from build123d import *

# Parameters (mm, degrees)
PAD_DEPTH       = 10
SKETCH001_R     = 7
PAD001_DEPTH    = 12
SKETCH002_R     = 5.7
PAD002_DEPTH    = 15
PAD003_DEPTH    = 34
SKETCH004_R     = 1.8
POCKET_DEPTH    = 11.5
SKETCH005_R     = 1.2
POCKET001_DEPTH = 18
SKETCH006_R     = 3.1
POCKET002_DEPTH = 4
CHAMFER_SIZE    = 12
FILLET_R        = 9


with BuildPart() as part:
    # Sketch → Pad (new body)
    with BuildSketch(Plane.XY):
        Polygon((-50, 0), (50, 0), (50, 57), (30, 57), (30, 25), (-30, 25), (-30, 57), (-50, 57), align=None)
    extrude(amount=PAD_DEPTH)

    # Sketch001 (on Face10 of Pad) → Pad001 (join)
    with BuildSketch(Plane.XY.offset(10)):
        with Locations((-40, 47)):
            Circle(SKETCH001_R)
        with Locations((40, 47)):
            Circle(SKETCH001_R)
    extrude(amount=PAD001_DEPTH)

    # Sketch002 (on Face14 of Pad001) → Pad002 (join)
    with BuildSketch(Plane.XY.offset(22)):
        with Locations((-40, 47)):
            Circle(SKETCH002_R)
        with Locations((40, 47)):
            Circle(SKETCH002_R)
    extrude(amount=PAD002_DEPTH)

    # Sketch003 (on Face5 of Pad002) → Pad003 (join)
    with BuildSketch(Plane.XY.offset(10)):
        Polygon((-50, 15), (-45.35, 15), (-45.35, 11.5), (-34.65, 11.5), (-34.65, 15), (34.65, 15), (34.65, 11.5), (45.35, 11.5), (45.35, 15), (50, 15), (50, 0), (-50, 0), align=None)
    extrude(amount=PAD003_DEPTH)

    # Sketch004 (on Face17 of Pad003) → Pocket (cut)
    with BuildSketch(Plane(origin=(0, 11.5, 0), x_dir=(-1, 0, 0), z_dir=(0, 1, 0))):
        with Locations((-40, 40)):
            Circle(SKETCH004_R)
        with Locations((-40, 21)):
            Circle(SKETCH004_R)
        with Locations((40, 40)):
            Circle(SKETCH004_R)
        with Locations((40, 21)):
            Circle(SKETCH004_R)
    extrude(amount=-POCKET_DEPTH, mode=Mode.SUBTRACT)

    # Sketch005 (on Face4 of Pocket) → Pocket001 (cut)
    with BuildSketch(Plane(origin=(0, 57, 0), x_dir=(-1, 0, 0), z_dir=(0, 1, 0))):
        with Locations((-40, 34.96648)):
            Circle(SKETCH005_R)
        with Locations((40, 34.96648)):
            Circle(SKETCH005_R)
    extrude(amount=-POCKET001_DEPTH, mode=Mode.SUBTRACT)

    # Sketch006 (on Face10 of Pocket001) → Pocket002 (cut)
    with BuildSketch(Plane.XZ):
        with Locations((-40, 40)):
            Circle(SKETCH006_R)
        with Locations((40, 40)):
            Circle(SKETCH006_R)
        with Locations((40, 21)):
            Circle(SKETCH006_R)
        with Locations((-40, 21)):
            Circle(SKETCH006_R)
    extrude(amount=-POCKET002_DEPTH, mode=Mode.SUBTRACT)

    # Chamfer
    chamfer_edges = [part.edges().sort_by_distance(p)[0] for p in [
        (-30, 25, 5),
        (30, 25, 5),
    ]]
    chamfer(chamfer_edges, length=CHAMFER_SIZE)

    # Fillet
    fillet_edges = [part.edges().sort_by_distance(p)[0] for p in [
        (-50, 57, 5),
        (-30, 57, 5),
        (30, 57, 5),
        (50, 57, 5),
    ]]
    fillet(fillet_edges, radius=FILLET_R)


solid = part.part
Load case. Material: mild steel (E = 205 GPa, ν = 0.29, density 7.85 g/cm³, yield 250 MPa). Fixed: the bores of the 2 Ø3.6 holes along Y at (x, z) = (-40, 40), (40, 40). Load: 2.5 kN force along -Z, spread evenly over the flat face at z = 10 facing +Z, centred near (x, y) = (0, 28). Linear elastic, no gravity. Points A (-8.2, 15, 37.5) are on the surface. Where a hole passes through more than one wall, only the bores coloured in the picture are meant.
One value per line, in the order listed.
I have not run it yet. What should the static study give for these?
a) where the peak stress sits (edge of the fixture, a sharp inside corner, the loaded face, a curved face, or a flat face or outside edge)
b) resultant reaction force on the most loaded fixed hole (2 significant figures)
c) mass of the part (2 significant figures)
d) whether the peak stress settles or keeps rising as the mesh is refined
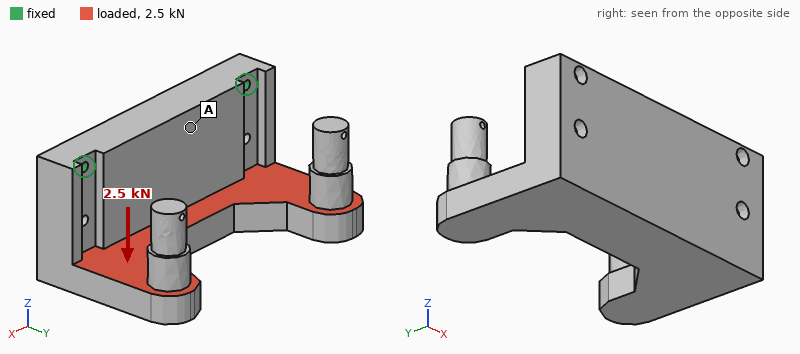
edge of the fixture
1.3 kN
730 g
keeps rising
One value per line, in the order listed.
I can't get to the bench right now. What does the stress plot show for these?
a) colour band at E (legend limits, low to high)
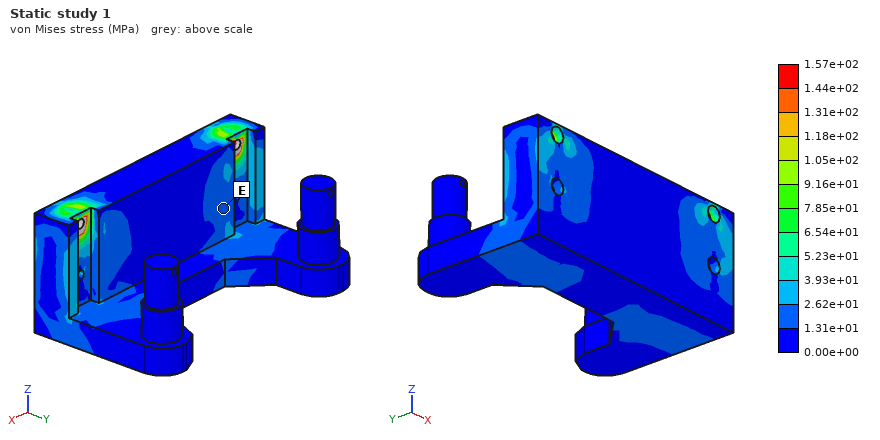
1.31e+01 to 2.62e+01 MPa
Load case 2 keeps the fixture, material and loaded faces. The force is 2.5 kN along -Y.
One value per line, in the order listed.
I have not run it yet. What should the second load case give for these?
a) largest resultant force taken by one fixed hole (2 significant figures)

1.3 kN
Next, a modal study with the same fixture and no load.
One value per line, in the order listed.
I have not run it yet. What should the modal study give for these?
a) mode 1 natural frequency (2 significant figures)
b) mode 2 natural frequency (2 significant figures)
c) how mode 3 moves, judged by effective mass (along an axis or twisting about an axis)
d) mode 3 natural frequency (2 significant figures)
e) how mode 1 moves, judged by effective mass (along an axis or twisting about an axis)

1300 Hz
2500 Hz
along Y
3200 Hz
along Y
